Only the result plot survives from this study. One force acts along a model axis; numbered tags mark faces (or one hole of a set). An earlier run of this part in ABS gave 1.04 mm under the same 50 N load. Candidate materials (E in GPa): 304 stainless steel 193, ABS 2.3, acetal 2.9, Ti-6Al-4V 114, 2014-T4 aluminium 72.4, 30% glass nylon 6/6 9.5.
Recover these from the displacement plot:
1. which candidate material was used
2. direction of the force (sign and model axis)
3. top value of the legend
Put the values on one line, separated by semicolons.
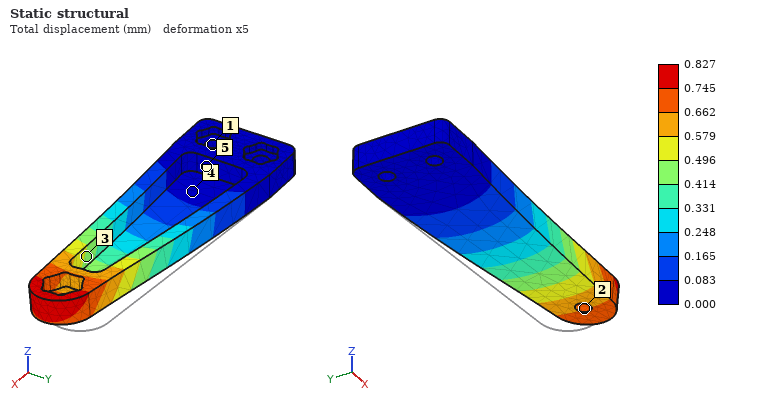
acetal; -Y; 0.827 mm
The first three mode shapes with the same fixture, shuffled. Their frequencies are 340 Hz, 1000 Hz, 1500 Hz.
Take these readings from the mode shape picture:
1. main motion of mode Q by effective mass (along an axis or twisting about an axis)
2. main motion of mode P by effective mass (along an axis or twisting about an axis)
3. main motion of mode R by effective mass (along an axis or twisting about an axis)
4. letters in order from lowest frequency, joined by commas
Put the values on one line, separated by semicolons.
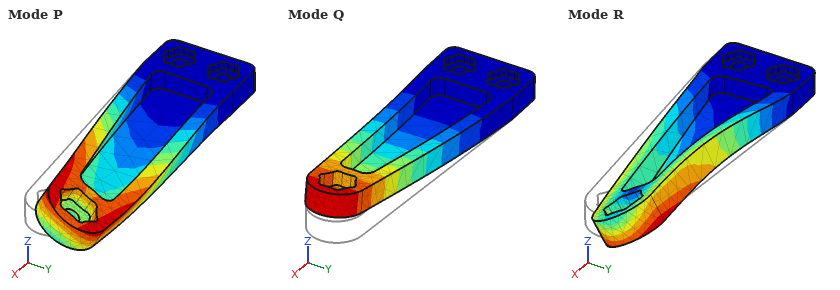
along Z; along Y; along Y; Q, P, R
